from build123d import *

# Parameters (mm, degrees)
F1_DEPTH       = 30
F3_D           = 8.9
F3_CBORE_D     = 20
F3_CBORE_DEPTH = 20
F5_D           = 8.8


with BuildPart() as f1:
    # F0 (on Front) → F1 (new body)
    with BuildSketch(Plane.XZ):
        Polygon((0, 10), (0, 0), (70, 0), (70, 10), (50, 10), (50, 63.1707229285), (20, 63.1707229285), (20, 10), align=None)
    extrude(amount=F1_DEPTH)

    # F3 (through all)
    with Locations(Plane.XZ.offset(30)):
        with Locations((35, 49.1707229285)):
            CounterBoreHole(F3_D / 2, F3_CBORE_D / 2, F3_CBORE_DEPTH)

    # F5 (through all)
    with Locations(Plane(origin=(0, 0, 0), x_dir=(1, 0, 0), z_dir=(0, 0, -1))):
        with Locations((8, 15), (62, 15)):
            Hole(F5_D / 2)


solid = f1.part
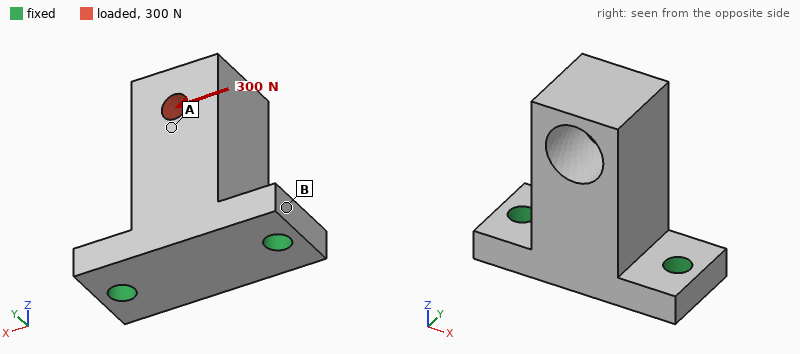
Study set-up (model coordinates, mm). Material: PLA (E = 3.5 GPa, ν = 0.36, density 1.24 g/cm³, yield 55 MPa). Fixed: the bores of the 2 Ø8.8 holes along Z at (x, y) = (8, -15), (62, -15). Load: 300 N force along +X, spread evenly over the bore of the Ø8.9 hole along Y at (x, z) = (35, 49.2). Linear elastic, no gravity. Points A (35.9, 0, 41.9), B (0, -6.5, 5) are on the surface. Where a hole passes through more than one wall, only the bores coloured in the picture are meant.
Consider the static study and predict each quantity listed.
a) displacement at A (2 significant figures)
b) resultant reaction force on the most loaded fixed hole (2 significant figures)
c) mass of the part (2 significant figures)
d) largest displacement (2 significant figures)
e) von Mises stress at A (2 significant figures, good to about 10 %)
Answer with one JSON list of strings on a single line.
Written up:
["0.087 mm", "360 N", "75 g", "0.15 mm", "2.7 MPa"]
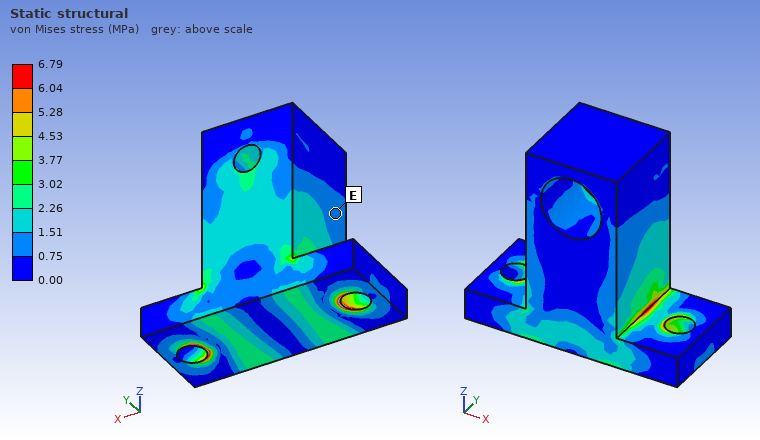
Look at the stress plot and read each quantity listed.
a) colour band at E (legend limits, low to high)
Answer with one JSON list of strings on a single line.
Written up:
["0.75 to 1.51 MPa"]
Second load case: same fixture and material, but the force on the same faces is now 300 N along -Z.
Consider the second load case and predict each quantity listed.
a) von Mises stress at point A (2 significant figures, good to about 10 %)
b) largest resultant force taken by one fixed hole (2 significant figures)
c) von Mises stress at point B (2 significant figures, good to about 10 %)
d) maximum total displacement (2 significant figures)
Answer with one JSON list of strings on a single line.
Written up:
["1.3 MPa", "160 N", "0.73 MPa", "0.12 mm"]
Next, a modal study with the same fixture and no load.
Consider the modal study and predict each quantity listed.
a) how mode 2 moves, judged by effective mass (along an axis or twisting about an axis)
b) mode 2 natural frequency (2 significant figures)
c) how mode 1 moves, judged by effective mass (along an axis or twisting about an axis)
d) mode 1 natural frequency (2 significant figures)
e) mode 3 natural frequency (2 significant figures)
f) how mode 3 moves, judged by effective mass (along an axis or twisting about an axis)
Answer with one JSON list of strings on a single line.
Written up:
["along X", "1600 Hz", "along Y", "830 Hz", "3000 Hz", "along Z"]
